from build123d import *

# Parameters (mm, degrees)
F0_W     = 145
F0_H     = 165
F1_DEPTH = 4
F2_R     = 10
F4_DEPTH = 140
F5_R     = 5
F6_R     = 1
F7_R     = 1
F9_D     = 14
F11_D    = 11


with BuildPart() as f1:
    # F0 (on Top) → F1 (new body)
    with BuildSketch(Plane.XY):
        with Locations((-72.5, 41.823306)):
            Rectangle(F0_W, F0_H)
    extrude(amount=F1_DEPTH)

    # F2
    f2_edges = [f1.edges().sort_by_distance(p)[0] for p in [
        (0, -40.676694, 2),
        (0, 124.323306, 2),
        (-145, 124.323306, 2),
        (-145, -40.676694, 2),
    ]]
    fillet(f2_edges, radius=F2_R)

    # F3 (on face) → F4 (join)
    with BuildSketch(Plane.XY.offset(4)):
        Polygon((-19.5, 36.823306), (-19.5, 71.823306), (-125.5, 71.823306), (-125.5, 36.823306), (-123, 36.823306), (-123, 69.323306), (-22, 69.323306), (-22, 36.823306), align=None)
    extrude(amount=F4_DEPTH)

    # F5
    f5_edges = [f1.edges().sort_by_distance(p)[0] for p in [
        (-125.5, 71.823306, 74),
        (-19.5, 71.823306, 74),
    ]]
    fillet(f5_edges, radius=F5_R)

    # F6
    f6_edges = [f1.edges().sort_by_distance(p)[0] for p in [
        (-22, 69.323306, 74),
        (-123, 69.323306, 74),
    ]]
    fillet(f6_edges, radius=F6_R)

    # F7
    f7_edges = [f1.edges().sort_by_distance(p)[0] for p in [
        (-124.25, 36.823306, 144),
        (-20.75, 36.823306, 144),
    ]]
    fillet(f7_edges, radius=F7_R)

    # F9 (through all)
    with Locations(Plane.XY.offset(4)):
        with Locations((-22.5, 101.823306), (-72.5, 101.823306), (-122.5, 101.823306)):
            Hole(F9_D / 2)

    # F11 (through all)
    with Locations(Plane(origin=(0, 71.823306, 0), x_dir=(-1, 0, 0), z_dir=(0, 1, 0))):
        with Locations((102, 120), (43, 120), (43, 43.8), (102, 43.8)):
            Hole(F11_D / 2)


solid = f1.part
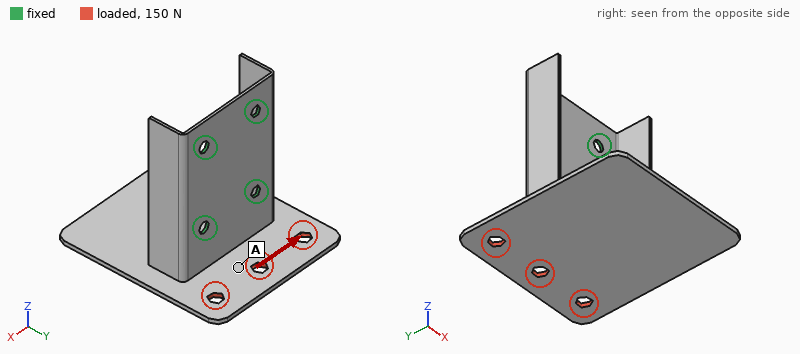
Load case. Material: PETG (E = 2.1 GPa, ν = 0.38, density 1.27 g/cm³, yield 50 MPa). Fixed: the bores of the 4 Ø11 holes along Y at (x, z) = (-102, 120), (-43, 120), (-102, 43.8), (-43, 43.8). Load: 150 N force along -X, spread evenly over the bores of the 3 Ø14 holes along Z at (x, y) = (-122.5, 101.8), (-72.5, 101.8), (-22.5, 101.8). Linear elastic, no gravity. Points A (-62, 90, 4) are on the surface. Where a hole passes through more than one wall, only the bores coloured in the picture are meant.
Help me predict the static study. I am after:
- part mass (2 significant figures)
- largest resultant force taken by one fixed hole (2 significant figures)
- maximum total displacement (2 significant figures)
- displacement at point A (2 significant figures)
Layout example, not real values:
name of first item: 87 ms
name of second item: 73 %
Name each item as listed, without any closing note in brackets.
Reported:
part mass: 190 g
largest resultant force taken by one fixed hole: 120 N
maximum total displacement: 3.1 mm
displacement at point A: 0.56 mm
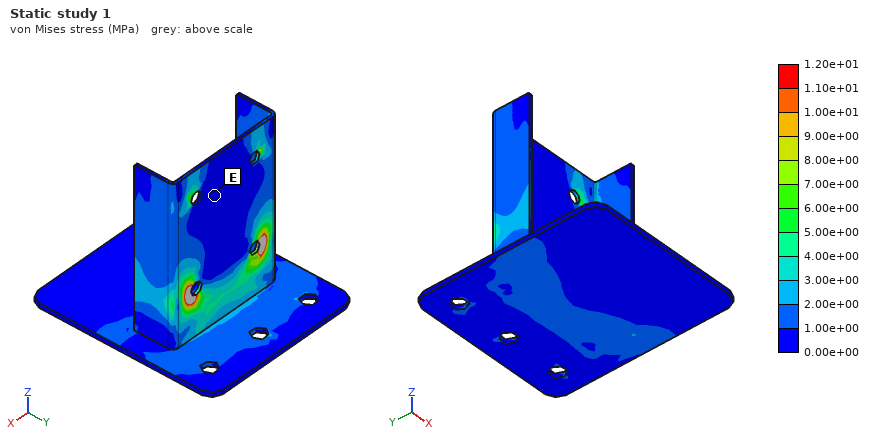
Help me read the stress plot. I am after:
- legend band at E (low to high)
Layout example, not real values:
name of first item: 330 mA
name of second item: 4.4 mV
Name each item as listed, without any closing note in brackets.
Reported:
legend band at E: 0.00e+00 to 1.00e+00 MPa
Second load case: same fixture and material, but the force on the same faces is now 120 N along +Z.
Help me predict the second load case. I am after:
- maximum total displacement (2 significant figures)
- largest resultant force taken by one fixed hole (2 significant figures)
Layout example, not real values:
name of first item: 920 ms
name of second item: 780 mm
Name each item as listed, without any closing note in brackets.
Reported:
maximum total displacement: 3.0 mm
largest resultant force taken by one fixed hole: 84 N
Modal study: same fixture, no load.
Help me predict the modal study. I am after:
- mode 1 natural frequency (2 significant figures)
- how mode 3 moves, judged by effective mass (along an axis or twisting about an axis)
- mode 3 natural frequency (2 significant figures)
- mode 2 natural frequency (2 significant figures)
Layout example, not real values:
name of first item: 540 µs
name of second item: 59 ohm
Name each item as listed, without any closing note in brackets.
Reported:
mode 1 natural frequency: 87 Hz
how mode 3 moves, judged by effective mass: along Y
mode 3 natural frequency: 150 Hz
mode 2 natural frequency: 87 Hz
